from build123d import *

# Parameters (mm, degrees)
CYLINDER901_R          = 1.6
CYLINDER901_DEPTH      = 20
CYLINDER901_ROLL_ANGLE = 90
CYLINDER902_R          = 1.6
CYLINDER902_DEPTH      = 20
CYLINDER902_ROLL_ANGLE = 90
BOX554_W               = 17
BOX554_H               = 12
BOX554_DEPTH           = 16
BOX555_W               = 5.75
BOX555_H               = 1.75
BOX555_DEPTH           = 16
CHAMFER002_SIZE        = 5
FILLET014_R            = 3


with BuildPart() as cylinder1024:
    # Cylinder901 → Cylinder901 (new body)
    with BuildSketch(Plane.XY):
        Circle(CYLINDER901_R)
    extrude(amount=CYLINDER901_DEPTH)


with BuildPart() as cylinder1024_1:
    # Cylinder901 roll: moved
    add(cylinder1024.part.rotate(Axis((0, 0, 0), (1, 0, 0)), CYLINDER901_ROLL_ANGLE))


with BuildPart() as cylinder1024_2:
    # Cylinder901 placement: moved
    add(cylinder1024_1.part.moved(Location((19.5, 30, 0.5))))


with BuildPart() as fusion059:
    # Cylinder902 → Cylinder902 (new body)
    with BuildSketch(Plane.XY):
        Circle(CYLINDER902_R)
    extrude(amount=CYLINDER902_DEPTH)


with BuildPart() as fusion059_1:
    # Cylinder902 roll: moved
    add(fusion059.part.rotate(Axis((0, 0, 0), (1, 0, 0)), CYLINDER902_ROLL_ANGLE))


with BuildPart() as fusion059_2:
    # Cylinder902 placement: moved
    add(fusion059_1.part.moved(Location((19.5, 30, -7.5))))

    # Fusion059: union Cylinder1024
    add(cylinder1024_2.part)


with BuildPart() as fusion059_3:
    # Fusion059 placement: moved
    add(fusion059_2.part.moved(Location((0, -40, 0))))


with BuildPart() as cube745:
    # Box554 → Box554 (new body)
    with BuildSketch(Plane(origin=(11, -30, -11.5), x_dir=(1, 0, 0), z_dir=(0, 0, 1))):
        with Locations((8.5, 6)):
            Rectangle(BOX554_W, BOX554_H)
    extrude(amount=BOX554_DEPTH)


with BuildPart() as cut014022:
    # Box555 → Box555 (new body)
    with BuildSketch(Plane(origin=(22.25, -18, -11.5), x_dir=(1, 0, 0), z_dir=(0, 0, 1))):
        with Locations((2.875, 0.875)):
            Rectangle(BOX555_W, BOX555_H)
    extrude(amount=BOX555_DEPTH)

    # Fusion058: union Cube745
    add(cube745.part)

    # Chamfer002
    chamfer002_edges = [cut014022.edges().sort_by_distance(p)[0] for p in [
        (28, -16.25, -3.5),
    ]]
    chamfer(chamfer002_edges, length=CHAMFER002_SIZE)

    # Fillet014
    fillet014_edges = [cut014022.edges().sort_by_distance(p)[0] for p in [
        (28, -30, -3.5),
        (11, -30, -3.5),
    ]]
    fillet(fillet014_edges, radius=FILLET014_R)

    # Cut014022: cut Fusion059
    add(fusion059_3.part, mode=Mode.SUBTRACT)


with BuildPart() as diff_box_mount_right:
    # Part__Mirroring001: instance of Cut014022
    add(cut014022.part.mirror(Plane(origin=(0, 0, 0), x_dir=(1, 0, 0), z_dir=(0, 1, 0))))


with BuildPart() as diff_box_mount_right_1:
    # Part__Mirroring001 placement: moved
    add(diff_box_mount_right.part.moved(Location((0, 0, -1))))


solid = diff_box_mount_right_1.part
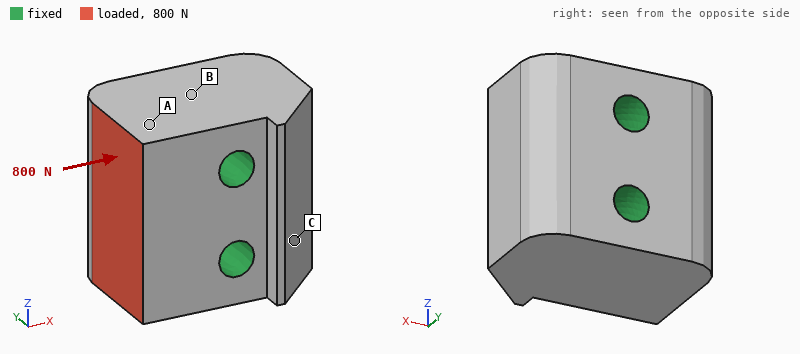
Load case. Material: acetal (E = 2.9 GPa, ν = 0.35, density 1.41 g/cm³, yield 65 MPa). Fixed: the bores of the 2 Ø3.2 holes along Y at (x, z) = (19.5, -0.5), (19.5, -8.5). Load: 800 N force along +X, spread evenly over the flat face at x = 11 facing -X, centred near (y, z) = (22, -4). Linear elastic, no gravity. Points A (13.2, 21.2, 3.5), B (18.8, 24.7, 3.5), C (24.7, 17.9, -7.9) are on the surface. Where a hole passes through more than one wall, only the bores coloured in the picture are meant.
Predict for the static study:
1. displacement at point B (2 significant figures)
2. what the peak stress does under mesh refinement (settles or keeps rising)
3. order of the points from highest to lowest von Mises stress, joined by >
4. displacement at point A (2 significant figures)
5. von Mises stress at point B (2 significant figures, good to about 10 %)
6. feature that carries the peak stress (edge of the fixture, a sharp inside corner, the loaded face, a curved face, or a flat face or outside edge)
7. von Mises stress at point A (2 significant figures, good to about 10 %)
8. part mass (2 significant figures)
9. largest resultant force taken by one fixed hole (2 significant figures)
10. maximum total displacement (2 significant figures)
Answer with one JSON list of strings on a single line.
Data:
["4.0 µm", "keeps rising", "A > B > C", "15 µm", "2.6 MPa", "edge of the fixture", "5.4 MPa", "4.2 g", "410 N", "22 µm"]
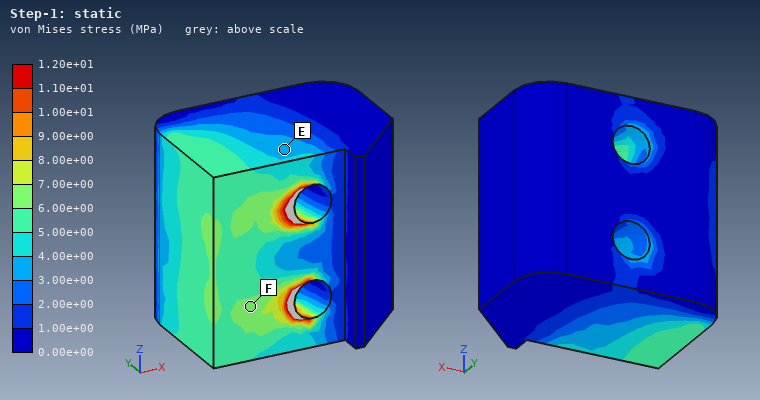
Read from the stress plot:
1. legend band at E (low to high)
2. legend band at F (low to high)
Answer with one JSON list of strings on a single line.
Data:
["3.00e+00 to 4.00e+00 MPa", "6.00e+00 to 7.00e+00 MPa"]
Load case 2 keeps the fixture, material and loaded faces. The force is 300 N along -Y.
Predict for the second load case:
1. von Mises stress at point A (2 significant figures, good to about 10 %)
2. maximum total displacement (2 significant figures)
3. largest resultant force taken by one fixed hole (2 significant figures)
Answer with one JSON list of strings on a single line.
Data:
["3.6 MPa", "28 µm", "150 N"]
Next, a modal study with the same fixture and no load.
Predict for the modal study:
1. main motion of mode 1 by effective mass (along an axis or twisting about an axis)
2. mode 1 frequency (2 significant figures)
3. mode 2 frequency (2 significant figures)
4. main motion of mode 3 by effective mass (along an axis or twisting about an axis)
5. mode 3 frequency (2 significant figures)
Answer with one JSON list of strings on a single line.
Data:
["twisting about Y", "21 kHz", "22 kHz", "along Y", "24 kHz"]
